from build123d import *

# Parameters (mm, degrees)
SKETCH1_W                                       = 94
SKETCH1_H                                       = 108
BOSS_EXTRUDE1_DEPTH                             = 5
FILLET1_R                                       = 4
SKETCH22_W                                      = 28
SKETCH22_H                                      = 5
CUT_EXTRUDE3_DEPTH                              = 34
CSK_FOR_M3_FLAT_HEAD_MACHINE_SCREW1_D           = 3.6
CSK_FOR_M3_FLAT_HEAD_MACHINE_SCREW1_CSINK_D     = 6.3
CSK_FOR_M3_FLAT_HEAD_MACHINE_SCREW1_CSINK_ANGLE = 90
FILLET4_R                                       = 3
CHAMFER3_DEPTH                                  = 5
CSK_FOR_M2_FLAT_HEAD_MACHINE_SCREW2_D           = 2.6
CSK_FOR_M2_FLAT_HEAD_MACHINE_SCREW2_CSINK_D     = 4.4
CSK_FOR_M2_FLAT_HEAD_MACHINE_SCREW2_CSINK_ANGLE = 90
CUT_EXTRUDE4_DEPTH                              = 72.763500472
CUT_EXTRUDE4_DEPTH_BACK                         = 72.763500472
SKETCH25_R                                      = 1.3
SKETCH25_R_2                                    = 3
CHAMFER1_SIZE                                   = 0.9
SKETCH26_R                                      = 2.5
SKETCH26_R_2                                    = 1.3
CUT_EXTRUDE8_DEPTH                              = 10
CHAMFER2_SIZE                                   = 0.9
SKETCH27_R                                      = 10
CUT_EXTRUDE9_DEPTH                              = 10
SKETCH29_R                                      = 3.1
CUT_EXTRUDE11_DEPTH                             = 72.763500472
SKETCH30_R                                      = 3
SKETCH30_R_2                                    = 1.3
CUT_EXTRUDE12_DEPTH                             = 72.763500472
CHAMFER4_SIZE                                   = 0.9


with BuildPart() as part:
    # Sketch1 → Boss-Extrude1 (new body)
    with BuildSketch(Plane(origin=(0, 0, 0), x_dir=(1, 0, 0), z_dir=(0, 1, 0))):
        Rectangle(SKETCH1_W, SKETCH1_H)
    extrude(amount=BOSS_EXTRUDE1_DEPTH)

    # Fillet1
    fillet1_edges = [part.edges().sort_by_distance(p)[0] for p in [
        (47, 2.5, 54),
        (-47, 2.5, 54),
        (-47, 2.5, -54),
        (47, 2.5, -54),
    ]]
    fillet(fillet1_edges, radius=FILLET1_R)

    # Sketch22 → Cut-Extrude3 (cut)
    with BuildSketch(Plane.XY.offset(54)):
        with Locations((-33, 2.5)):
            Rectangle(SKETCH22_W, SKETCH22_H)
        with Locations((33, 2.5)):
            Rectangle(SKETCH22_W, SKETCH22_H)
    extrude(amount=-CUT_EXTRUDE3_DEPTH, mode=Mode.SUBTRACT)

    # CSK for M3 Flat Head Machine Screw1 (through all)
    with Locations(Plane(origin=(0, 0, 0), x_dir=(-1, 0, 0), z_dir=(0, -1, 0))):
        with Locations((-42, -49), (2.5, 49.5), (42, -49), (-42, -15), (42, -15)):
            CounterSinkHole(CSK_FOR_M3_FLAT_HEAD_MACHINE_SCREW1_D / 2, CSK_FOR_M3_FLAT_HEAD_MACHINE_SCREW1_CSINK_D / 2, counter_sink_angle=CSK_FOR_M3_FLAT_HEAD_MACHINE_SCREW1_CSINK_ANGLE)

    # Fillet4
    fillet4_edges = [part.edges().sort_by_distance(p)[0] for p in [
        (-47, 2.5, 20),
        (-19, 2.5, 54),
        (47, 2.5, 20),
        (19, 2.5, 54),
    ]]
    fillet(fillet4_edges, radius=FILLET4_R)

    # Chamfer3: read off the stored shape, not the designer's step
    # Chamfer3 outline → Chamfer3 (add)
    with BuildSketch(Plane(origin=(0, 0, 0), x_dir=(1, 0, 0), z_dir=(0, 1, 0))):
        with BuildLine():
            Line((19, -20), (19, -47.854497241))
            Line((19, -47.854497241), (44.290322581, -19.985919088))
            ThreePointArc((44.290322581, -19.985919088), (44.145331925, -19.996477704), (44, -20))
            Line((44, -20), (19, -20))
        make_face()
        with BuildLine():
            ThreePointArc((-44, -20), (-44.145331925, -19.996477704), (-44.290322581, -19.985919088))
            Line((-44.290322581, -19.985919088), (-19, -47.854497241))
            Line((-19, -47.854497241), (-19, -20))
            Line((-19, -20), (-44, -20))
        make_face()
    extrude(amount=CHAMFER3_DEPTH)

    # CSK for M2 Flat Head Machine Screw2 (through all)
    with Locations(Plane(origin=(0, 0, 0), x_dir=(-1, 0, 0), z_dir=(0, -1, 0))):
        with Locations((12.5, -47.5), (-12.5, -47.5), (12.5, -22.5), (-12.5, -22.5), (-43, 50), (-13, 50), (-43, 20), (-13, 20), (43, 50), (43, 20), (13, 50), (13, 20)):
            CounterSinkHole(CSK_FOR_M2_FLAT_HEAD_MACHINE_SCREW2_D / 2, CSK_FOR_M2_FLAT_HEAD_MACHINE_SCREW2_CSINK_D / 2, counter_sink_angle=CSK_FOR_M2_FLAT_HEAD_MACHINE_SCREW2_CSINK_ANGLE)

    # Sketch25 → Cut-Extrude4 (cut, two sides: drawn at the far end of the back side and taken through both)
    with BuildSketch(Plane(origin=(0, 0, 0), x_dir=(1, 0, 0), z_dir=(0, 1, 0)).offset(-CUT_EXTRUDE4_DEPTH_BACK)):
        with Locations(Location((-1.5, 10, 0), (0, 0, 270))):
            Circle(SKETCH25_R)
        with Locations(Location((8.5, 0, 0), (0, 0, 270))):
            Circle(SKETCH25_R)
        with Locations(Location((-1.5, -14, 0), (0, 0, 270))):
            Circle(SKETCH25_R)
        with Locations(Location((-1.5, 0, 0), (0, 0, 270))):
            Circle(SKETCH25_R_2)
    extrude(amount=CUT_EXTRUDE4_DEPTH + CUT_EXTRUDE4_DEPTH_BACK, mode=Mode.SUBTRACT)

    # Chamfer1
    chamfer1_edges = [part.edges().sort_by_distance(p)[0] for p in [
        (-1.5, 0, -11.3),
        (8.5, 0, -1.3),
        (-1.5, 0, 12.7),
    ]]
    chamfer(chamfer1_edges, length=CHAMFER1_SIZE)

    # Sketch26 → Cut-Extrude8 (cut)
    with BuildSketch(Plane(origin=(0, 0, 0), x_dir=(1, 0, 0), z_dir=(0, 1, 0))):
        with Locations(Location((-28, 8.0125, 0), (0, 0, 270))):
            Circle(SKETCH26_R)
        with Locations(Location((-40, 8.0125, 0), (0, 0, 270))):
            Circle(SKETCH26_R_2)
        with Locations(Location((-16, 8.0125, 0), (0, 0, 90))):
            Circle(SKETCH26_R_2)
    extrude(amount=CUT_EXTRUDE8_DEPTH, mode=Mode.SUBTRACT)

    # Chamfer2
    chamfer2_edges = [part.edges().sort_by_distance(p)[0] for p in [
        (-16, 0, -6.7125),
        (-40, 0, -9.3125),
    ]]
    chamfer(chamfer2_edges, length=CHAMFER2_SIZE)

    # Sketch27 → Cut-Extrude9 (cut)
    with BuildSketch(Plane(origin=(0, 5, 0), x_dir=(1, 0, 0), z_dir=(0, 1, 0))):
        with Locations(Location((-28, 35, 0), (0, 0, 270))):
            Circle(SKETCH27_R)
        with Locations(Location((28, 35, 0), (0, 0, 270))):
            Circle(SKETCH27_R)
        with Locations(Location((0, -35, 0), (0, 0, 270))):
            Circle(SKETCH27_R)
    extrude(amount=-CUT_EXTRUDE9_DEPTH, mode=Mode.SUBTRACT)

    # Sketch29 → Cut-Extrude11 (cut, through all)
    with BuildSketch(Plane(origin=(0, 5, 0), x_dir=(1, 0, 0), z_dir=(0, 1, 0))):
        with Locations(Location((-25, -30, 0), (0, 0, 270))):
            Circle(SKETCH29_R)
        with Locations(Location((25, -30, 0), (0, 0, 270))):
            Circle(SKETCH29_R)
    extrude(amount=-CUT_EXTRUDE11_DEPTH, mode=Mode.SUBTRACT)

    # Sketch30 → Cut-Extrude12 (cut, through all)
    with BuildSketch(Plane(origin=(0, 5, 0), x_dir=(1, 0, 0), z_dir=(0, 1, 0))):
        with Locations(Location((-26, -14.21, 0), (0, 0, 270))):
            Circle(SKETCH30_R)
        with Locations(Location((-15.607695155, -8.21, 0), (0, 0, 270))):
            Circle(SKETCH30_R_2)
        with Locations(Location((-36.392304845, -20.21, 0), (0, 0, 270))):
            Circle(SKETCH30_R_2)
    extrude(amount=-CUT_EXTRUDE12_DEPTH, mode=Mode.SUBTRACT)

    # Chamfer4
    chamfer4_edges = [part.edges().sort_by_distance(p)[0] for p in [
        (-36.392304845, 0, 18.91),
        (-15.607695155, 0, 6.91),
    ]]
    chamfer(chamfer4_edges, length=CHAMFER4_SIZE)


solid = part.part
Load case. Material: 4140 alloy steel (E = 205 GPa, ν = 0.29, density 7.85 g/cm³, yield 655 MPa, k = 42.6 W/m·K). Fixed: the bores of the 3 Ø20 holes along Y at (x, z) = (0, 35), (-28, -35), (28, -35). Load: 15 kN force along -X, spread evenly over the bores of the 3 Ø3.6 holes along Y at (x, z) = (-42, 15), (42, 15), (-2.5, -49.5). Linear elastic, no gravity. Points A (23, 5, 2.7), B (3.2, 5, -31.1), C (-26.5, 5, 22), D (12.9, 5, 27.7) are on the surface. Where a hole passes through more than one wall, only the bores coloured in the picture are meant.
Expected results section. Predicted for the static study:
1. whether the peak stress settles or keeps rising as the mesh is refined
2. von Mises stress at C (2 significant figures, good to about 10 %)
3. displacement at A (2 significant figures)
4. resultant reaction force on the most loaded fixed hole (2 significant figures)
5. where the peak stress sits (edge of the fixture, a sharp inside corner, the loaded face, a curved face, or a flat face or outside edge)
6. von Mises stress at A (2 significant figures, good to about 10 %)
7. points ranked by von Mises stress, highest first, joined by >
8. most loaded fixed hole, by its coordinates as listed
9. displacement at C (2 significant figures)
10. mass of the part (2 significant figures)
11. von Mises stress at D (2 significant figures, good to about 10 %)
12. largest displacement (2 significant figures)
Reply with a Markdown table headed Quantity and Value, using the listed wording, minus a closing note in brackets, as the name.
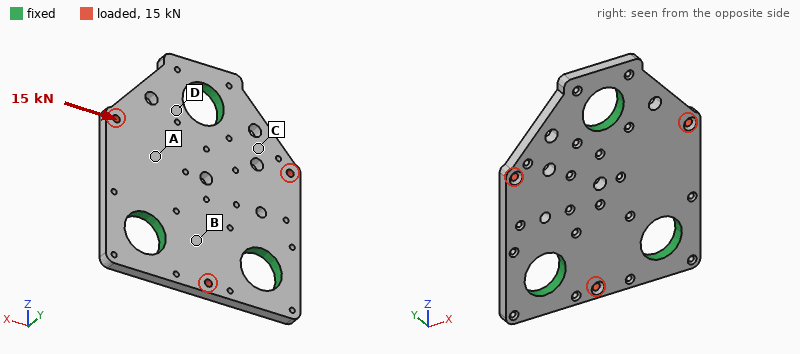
| Quantity | Value |
|---|---|
| whether the peak stress settles or keeps rising as the mesh is refined | keeps rising |
| von Mises stress at C | 60 MPa |
| displacement at A | 4.7 µm |
| resultant reaction force on the most loaded fixed hole | 6.7 kN |
| where the peak stress sits | a sharp inside corner |
| von Mises stress at A | 27 MPa |
| points ranked by von Mises stress, highest first, joined by > | C > D > A > B |
| most loaded fixed hole, by its coordinates as listed | (0, 35) |
| displacement at C | 6.2 µm |
| mass of the part | 300 g |
| von Mises stress at D | 47 MPa |
| largest displacement | 25 µm |
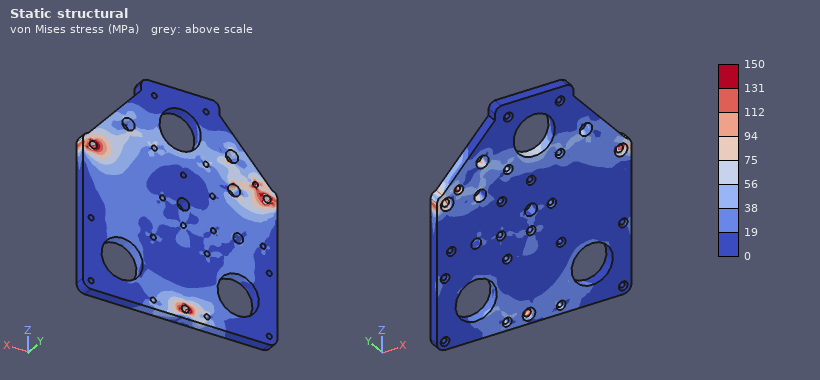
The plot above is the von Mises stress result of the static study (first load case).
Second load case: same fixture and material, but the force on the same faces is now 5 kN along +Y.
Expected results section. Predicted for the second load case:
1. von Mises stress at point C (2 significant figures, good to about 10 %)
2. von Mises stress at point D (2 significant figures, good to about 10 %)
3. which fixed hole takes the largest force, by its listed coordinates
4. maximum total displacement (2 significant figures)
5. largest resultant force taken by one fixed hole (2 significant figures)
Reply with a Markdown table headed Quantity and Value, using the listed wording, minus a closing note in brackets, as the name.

| Quantity | Value |
|---|---|
| von Mises stress at point C | 120 MPa |
| von Mises stress at point D | 150 MPa |
| which fixed hole takes the largest force, by its listed coordinates | (0, 35) |
| maximum total displacement | 0.20 mm |
| largest resultant force taken by one fixed hole | 2.0 kN |
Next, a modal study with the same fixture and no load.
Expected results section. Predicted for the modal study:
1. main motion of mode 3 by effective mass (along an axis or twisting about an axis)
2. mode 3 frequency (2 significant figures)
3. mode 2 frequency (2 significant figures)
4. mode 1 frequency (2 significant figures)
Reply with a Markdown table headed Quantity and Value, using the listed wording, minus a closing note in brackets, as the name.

| Quantity | Value |
|---|---|
| main motion of mode 3 by effective mass | along Y |
| mode 3 frequency | 8100 Hz |
| mode 2 frequency | 4400 Hz |
| mode 1 frequency | 4300 Hz |
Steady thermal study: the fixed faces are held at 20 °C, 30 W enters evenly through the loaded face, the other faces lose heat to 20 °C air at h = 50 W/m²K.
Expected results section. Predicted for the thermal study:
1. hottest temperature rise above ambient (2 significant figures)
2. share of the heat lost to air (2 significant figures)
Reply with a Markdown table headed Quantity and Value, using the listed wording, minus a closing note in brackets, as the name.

| Quantity | Value |
|---|---|
| hottest temperature rise above ambient | 50 K |
| share of the heat lost to air | 26 % |
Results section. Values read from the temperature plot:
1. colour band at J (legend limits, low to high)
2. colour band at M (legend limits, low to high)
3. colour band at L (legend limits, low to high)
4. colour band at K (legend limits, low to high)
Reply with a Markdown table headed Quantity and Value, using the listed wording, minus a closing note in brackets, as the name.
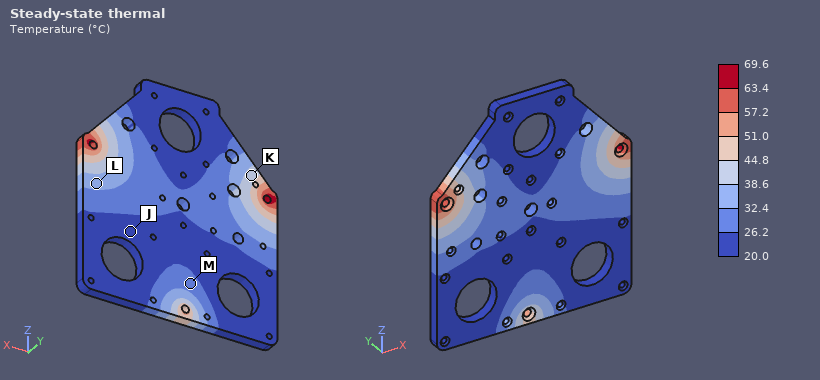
| Quantity | Value |
|---|---|
| colour band at J | 20.0 to 26.2 °C |
| colour band at M | 26.2 to 32.4 °C |
| colour band at L | 32.4 to 38.6 °C |
| colour band at K | 38.6 to 44.8 °C |
